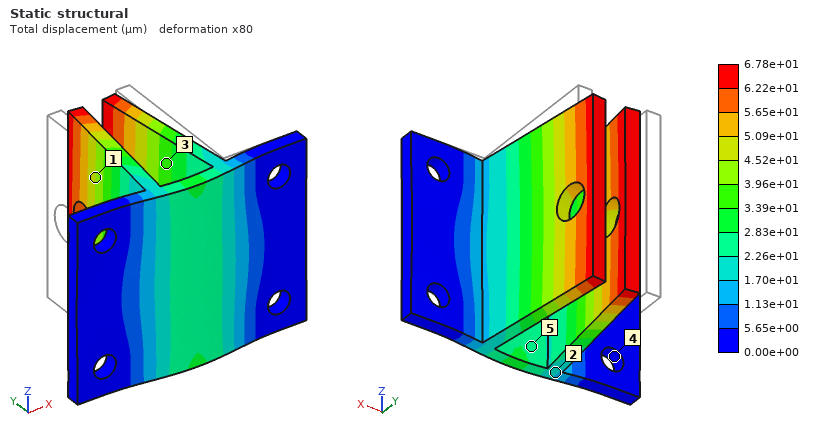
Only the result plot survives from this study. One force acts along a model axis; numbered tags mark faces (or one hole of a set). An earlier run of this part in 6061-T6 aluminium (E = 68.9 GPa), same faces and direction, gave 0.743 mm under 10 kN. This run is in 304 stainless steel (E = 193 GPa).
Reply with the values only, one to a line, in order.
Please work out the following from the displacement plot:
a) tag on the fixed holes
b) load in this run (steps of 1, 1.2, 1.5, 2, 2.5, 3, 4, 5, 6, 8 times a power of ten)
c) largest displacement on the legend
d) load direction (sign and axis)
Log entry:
4
2.5 kN
6.78e+01 µm
-Y
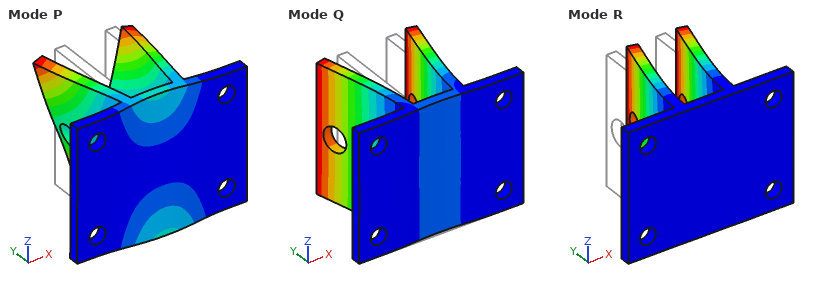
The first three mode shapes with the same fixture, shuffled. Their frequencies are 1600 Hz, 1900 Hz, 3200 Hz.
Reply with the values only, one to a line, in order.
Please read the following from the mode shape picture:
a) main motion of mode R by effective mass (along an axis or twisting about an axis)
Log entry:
along X
